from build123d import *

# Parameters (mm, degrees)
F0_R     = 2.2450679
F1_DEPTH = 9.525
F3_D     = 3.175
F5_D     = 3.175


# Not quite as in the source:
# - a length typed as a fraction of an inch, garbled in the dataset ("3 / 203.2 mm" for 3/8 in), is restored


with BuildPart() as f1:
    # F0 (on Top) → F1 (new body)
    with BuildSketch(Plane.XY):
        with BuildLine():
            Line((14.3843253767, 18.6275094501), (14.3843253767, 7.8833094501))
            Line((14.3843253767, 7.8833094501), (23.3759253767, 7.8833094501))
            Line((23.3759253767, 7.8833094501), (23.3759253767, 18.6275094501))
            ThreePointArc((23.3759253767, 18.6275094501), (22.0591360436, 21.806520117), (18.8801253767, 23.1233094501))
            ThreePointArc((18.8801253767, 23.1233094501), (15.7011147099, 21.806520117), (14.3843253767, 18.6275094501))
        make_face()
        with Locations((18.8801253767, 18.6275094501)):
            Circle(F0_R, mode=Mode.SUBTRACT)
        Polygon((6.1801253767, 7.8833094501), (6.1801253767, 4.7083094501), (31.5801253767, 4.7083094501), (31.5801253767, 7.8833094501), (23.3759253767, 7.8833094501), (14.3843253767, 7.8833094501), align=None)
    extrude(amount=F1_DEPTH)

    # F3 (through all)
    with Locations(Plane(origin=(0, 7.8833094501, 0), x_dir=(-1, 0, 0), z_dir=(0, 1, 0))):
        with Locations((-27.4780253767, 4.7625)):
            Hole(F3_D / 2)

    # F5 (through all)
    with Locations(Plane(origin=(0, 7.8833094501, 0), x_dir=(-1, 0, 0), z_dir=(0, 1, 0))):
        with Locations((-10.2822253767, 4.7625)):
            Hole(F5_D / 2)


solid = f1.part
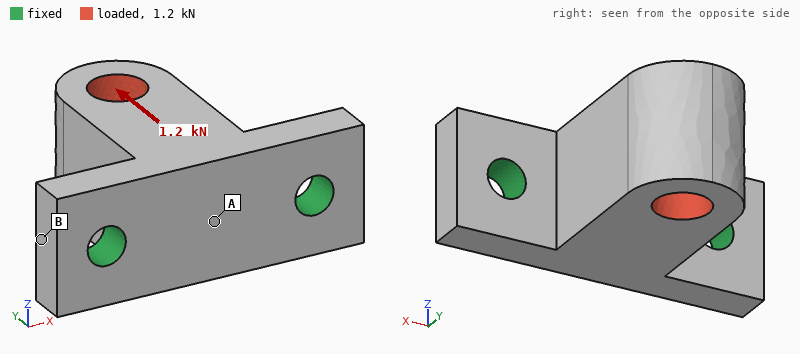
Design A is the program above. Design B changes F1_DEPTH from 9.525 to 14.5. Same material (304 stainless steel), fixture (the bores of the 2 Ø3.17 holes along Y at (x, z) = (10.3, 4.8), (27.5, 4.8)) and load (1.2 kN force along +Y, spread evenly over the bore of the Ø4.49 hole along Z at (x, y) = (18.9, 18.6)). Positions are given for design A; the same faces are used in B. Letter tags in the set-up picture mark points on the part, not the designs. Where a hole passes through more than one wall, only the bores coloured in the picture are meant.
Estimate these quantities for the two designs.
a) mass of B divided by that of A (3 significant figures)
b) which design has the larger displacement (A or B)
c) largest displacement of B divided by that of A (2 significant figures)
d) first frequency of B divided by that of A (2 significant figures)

1.54
B
2.9
0.87
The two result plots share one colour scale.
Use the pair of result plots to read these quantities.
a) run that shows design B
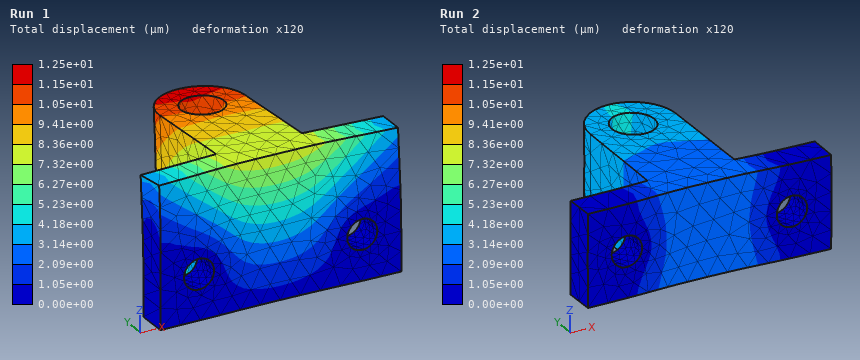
Run 1
